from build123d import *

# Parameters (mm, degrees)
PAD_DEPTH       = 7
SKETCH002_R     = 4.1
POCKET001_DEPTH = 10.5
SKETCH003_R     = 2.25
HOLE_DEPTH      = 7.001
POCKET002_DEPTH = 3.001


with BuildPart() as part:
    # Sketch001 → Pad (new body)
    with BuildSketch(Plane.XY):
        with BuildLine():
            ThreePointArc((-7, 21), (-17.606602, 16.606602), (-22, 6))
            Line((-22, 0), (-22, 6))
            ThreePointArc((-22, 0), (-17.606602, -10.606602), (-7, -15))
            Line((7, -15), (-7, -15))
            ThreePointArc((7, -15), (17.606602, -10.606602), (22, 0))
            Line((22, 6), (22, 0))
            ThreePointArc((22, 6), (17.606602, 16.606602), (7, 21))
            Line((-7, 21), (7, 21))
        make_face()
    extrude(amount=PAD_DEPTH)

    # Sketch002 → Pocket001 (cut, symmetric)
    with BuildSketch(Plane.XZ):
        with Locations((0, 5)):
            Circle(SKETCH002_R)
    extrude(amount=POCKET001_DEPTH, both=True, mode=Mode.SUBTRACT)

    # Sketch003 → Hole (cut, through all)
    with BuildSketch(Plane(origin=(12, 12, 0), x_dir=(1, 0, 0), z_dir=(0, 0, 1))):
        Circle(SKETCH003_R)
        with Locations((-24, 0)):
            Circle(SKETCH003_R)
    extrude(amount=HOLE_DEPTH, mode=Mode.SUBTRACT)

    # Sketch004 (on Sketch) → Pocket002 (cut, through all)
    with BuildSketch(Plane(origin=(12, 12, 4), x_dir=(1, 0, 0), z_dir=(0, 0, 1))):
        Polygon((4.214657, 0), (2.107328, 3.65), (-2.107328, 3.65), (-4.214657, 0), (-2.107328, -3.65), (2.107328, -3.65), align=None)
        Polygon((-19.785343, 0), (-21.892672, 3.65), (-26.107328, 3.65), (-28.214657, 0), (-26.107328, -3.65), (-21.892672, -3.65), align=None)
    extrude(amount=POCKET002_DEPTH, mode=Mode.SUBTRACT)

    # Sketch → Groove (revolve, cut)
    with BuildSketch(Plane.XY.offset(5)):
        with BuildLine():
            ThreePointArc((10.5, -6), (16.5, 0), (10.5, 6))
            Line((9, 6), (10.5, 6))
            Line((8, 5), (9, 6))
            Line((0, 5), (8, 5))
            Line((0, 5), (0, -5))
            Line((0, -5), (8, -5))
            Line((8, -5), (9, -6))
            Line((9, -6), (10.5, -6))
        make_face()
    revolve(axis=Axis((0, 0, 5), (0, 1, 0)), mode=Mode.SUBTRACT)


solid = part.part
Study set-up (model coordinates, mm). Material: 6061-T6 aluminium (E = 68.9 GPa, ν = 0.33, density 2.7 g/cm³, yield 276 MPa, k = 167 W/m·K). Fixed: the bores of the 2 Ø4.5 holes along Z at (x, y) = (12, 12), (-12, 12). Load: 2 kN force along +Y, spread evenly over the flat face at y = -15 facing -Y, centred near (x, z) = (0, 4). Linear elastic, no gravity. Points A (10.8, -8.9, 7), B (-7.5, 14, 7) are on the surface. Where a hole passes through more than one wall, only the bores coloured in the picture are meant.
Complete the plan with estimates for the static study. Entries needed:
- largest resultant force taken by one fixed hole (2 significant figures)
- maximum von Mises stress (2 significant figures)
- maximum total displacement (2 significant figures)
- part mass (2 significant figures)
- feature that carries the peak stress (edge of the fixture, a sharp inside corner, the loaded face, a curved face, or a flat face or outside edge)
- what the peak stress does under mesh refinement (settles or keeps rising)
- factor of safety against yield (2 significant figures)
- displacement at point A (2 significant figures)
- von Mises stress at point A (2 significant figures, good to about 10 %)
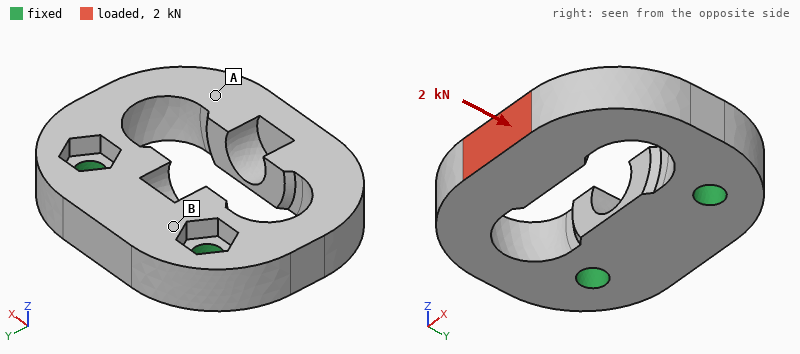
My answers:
1.2 kN
430 MPa
82 µm
18 g
a curved face
settles
0.65
47 µm
43 MPa
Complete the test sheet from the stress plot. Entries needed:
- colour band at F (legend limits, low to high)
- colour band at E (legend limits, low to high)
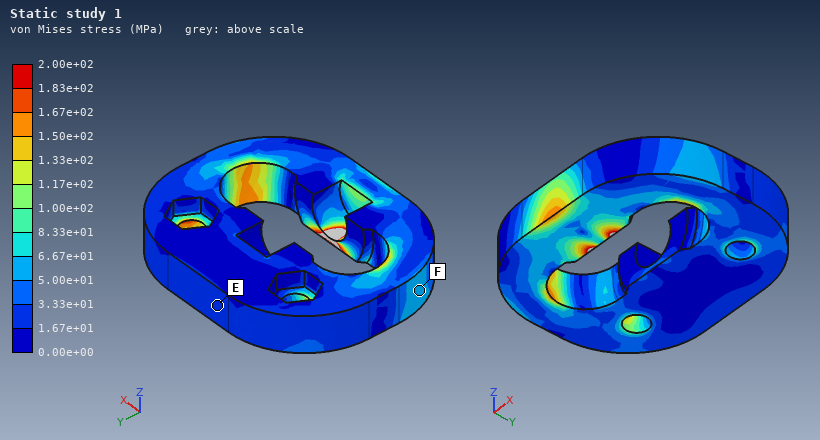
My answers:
5.00e+01 to 6.67e+01 MPa
1.67e+01 to 3.33e+01 MPa
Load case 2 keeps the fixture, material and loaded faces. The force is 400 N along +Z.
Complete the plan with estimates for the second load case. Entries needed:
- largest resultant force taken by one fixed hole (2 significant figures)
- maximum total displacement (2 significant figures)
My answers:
230 N
0.17 mm
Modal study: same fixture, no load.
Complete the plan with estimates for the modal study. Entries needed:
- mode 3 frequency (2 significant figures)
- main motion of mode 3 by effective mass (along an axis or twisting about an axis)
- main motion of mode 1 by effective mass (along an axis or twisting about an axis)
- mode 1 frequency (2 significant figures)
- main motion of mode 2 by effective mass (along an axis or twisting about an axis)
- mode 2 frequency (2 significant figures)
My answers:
9700 Hz
along X
along Z
4300 Hz
along X
9300 Hz
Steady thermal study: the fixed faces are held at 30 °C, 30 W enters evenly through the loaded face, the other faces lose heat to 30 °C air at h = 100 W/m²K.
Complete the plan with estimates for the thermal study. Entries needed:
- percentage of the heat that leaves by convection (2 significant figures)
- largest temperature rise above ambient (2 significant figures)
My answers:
22 %
58 K
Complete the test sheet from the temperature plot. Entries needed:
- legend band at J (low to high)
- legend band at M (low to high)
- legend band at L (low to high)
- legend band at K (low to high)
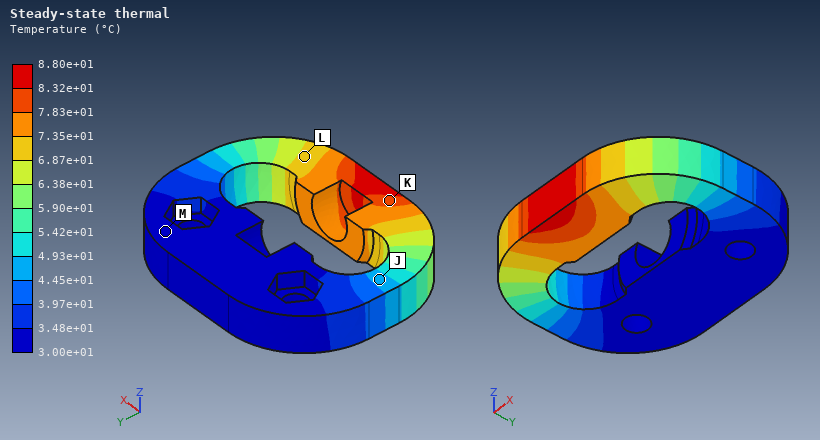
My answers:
4.45e+01 to 4.93e+01 °C
3.00e+01 to 3.48e+01 °C
6.87e+01 to 7.35e+01 °C
7.83e+01 to 8.32e+01 °C
